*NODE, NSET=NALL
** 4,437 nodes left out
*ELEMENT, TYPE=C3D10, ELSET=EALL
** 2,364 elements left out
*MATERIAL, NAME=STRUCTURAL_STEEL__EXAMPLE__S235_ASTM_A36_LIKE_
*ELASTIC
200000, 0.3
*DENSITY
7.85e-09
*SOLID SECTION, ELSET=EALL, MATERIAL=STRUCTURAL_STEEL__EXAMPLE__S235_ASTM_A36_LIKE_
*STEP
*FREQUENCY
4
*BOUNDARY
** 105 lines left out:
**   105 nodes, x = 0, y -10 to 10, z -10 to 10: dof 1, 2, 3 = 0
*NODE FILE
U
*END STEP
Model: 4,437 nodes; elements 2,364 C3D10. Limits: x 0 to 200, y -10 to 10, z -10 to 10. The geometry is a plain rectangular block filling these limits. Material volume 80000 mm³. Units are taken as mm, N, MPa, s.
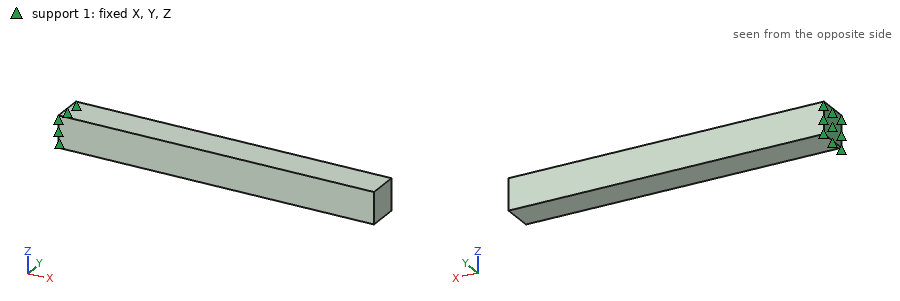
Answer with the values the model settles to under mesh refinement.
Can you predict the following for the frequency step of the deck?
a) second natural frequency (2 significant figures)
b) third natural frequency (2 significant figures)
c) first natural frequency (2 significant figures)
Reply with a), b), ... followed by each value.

a) 410 Hz
b) 2400 Hz
c) 410 Hz
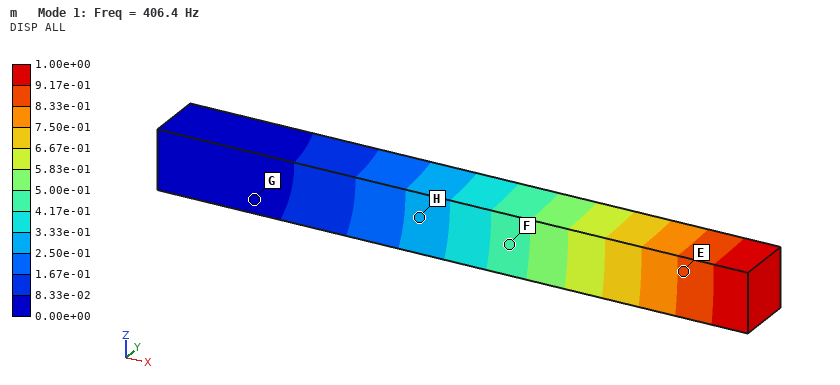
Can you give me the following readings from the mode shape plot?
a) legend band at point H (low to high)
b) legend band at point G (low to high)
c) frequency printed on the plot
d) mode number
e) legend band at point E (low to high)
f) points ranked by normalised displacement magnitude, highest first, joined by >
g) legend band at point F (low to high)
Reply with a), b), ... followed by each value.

a) 2.50e-01 to 3.33e-01
b) 0.00e+00 to 8.33e-02
c) 406.4 Hz
d) 1
e) 8.33e-01 to 9.17e-01
f) E > F > H > G
g) 4.17e-01 to 5.00e-01
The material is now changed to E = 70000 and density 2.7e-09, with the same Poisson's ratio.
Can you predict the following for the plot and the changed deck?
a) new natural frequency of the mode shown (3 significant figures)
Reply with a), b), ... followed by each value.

a) 410 Hz
